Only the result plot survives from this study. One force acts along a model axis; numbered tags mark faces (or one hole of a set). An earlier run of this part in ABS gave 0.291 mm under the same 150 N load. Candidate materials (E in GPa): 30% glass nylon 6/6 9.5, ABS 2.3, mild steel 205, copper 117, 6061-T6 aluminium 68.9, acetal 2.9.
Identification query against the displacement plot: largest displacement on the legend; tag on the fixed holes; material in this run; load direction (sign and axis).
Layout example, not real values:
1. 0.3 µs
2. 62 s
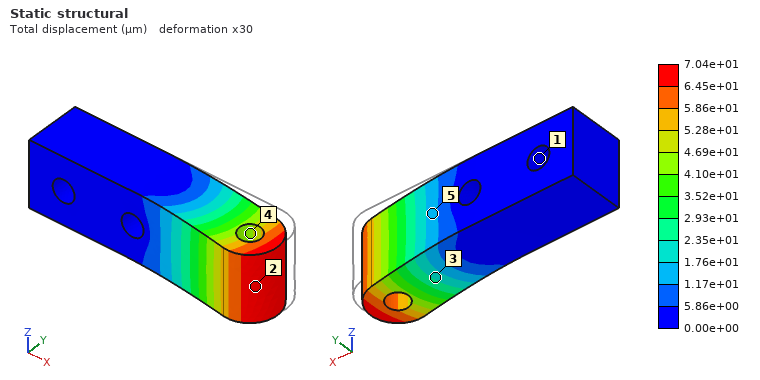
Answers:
1. 7.04e+01 µm
2. 1
3. 30% glass nylon 6/6
4. -Y
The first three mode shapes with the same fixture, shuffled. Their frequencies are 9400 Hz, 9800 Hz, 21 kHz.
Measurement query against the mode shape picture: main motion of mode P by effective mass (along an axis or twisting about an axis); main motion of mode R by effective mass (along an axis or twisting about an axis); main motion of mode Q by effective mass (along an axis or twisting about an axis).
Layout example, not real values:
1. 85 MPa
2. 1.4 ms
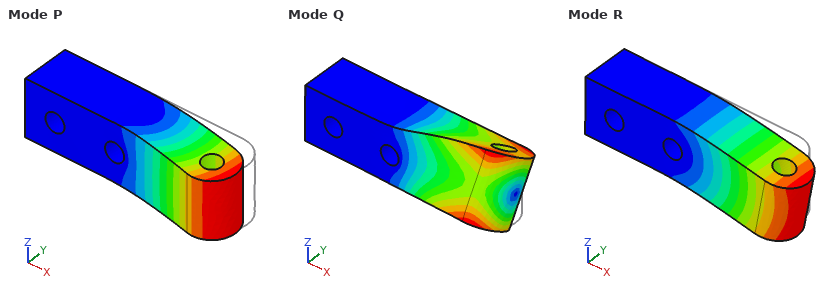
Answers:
1. along Y
2. along Z
3. twisting about X
